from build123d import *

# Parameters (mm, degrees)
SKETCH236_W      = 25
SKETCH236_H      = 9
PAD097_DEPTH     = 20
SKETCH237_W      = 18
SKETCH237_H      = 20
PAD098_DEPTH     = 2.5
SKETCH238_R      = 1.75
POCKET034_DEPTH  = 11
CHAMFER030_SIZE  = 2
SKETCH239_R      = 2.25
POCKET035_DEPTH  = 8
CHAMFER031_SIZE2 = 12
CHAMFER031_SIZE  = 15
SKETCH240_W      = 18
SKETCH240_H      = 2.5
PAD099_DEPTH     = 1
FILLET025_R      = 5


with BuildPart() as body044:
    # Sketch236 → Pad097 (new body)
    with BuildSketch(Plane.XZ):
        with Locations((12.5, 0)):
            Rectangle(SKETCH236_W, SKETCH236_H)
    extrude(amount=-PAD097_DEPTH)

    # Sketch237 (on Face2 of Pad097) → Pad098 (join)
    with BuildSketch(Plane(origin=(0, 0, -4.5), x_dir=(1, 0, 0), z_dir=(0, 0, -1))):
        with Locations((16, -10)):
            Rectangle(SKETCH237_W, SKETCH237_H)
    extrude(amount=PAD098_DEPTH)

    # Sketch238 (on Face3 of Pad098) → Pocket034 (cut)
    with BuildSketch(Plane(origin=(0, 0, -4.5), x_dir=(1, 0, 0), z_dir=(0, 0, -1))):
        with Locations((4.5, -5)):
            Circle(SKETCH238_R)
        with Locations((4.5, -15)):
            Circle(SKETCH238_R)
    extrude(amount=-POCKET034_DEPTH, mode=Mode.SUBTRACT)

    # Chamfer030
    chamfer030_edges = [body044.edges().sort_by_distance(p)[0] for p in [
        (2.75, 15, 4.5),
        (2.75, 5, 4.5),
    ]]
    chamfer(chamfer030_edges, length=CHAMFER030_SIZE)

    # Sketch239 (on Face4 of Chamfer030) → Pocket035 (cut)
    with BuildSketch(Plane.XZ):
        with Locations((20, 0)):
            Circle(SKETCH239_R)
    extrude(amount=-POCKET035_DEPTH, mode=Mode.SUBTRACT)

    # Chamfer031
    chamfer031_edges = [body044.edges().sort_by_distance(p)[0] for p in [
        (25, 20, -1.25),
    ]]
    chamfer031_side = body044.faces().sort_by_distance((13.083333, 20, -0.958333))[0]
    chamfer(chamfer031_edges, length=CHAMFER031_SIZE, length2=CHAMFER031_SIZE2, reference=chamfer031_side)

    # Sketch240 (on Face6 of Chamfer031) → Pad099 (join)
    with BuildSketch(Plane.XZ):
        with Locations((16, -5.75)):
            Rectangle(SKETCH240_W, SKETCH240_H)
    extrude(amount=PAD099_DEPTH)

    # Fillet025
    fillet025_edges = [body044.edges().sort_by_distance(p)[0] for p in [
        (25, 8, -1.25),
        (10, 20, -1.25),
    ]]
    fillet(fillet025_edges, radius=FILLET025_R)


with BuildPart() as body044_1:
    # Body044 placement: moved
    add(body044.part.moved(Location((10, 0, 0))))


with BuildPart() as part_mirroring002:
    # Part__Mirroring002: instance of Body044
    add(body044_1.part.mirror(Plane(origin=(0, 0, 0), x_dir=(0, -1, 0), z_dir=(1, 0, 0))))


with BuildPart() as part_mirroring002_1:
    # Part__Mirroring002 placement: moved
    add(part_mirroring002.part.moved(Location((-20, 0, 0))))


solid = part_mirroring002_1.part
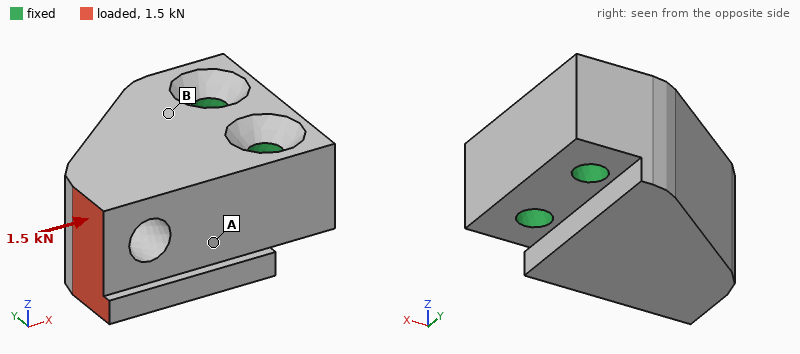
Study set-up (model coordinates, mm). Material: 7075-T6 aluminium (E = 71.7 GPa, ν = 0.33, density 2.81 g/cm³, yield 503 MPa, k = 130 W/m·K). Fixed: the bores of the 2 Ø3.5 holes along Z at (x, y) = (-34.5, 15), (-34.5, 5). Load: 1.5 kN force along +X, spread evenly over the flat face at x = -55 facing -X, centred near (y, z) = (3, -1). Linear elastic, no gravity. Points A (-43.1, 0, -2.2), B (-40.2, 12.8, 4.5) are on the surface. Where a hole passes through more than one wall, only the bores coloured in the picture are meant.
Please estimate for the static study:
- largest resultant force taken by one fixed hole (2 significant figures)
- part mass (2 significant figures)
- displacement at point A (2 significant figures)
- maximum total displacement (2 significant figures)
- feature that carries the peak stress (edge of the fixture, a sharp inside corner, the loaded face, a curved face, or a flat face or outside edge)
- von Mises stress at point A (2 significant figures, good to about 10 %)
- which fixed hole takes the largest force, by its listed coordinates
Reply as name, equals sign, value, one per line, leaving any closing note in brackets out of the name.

largest resultant force taken by one fixed hole = 1.7 kN
part mass = 11 g
displacement at point A = 4.4 µm
maximum total displacement = 14 µm
feature that carries the peak stress = a curved face
von Mises stress at point A = 24 MPa
which fixed hole takes the largest force, by its listed coordinates = (-34.5, 5)
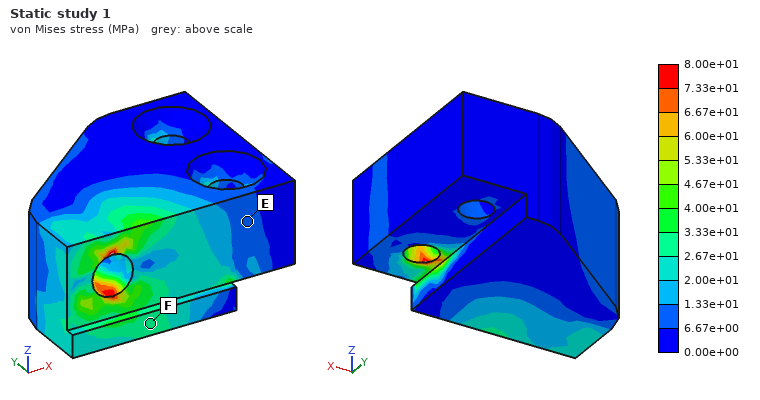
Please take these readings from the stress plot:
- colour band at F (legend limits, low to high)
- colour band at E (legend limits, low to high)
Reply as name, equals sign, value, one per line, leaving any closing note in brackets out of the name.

colour band at F = 2.67e+01 to 3.33e+01 MPa
colour band at E = 6.67e+00 to 1.33e+01 MPa
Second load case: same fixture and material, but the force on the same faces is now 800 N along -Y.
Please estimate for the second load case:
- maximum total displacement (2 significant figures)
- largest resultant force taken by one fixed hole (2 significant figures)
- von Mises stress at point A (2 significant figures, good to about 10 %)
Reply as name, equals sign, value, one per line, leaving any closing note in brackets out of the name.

maximum total displacement = 17 µm
largest resultant force taken by one fixed hole = 1.4 kN
von Mises stress at point A = 19 MPa
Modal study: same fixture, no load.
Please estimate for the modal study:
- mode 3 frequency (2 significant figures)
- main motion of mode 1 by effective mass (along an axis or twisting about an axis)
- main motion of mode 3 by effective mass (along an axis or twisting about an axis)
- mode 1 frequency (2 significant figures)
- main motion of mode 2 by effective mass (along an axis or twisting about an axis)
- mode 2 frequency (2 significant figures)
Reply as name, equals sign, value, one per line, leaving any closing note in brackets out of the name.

mode 3 frequency = 41 kHz
main motion of mode 1 by effective mass = along Z
main motion of mode 3 by effective mass = twisting about X
mode 1 frequency = 16 kHz
main motion of mode 2 by effective mass = along Y
mode 2 frequency = 27 kHz
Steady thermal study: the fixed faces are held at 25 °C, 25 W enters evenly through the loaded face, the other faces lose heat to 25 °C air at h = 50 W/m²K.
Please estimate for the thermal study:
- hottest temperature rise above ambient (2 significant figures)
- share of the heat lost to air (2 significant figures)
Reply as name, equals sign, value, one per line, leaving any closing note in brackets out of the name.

hottest temperature rise above ambient = 36 K
share of the heat lost to air = 3.2 %
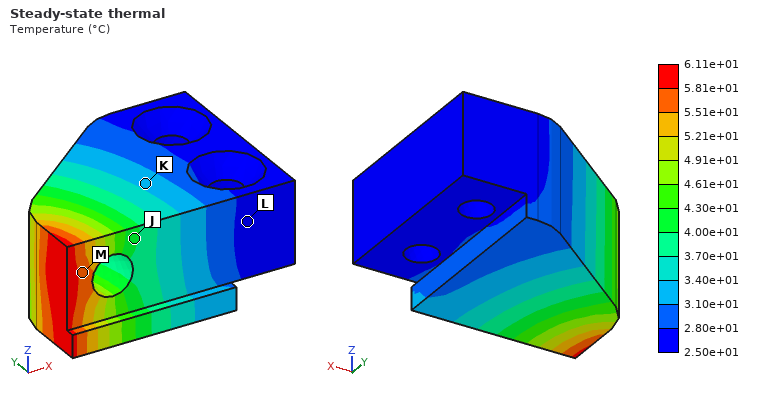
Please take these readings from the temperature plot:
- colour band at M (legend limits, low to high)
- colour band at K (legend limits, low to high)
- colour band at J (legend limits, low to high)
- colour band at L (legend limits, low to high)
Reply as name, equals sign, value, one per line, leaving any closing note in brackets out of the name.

colour band at M = 5.51e+01 to 5.81e+01 °C
colour band at K = 3.10e+01 to 3.40e+01 °C
colour band at J = 4.00e+01 to 4.30e+01 °C
colour band at L = 2.50e+01 to 2.80e+01 °C
